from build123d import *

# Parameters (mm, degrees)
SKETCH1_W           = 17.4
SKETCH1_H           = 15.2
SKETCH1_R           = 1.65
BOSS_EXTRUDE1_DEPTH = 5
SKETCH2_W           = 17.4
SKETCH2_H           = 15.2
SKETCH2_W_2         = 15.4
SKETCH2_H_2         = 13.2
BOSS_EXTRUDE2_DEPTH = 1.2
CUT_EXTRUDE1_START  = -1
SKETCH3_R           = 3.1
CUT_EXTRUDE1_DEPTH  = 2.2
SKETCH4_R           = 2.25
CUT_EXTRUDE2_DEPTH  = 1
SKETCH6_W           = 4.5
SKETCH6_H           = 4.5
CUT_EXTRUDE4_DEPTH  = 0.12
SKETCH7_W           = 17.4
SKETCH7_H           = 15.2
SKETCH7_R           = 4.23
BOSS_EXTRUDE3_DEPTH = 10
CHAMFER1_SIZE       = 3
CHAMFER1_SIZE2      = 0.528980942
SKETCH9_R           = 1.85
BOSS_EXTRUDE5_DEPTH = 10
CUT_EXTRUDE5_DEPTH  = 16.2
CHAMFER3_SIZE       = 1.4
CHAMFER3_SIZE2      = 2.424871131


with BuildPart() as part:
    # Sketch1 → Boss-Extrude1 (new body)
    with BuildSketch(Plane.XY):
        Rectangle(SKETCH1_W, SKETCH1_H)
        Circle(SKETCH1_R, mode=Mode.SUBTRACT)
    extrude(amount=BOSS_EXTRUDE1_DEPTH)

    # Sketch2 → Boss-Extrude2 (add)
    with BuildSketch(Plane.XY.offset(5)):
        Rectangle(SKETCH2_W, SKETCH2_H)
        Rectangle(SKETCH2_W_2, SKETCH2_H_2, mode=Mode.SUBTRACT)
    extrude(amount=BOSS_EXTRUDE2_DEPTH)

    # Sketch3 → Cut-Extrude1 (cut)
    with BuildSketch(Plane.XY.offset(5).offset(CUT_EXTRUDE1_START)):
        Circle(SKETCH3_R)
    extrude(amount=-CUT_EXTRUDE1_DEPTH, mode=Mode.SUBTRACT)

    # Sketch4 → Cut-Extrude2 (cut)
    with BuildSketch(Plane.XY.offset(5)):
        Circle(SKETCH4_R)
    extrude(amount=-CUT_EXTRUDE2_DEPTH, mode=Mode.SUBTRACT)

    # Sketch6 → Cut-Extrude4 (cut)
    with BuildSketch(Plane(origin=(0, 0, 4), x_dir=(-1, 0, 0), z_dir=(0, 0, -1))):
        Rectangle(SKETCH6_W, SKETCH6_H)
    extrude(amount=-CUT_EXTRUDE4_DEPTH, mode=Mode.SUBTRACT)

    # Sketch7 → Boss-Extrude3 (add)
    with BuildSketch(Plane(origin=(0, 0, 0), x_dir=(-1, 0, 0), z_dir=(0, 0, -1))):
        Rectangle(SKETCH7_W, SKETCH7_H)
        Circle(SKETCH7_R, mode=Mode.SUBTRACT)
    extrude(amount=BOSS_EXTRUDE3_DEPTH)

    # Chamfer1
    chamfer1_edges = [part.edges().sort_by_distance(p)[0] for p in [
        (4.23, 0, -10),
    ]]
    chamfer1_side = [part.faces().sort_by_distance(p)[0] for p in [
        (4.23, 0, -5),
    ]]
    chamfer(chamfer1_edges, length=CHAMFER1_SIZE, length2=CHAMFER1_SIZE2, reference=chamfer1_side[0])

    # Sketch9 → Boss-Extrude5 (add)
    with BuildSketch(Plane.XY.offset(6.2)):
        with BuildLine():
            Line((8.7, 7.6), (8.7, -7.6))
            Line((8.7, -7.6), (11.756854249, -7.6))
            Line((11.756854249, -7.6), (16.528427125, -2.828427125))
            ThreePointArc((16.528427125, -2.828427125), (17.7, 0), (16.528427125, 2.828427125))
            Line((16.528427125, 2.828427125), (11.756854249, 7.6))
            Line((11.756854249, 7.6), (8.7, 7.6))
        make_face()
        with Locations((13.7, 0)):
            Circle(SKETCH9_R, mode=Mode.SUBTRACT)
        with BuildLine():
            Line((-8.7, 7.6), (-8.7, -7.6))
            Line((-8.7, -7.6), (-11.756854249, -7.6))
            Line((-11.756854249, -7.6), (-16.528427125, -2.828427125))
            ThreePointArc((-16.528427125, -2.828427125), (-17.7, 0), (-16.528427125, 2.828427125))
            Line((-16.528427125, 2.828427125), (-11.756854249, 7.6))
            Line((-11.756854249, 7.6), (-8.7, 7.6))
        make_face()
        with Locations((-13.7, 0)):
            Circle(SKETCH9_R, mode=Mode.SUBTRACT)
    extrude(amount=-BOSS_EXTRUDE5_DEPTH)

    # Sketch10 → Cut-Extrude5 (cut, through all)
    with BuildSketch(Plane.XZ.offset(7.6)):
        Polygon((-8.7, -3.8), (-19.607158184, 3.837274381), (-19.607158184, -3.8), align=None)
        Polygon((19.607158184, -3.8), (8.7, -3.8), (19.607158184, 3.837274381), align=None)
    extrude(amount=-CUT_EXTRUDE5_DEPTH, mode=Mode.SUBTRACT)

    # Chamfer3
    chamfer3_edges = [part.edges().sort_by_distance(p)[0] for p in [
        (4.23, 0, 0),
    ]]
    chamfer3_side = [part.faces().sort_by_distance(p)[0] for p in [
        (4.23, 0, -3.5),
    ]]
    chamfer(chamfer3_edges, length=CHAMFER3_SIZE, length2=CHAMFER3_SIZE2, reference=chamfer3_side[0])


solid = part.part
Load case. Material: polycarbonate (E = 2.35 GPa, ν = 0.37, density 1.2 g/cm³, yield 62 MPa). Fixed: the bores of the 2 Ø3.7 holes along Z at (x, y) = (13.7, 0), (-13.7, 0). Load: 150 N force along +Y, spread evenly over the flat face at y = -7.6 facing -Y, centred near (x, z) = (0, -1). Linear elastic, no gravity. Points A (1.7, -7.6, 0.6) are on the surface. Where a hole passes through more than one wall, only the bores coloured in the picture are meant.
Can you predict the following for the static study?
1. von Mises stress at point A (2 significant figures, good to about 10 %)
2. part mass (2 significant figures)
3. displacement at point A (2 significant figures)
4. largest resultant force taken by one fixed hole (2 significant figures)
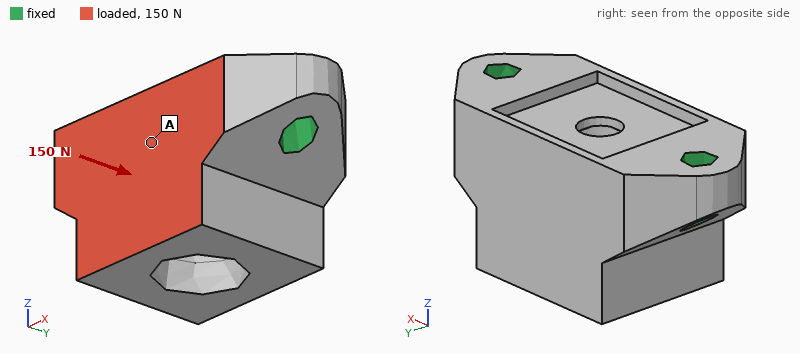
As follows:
1.4 MPa
5.7 g
16 µm
76 N
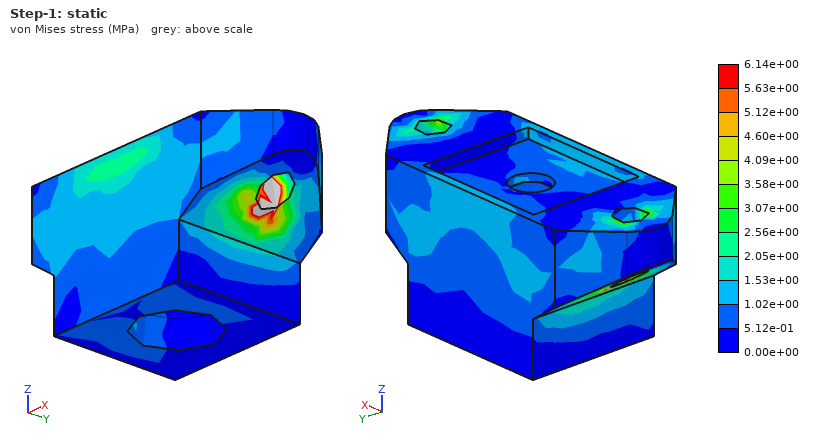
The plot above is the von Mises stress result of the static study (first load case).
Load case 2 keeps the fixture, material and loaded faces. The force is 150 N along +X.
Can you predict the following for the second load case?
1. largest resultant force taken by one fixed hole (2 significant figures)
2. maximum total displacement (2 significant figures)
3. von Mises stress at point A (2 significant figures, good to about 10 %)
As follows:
87 N
13 µm
1.0 MPa
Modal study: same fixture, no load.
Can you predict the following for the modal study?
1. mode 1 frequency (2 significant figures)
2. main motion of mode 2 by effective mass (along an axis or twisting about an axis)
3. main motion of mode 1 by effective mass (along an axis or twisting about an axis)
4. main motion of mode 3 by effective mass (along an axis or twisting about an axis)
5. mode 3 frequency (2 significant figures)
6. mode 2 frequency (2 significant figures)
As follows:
5800 Hz
along Z
along Y
along Y
12 kHz
9400 Hz
